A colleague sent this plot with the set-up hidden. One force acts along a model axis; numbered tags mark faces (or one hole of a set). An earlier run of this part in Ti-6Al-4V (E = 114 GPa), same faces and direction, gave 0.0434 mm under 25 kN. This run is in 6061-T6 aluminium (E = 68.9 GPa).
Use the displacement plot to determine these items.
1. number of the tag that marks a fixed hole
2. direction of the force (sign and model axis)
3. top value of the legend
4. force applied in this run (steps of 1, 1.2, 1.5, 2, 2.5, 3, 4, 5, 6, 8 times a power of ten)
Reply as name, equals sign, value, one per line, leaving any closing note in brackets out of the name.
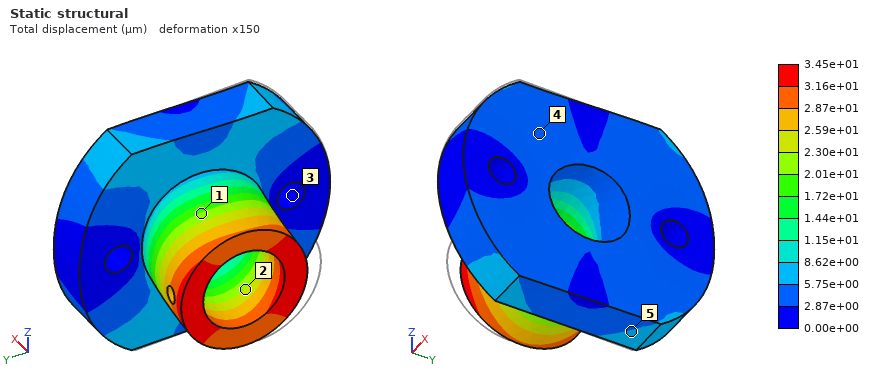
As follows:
number of the tag that marks a fixed hole = 3
direction of the force = +Y
top value of the legend = 3.45e+01 µm
force applied in this run = 12 kN
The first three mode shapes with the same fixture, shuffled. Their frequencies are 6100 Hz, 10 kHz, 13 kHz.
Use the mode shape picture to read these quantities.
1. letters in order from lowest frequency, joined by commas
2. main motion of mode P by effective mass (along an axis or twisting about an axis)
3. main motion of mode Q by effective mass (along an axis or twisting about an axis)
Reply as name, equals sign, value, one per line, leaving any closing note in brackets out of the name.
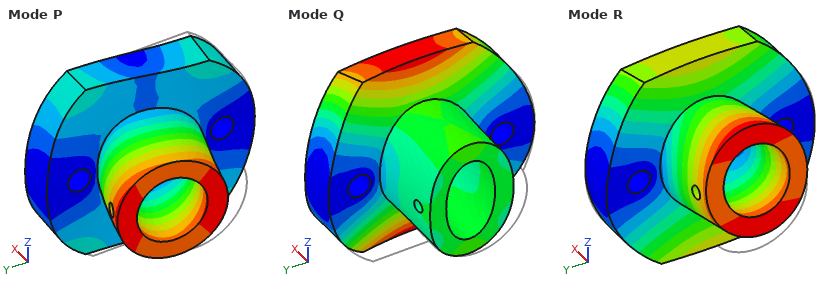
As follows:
letters in order from lowest frequency, joined by commas = R, Q, P
main motion of mode P by effective mass = along Y
main motion of mode Q by effective mass = along X
